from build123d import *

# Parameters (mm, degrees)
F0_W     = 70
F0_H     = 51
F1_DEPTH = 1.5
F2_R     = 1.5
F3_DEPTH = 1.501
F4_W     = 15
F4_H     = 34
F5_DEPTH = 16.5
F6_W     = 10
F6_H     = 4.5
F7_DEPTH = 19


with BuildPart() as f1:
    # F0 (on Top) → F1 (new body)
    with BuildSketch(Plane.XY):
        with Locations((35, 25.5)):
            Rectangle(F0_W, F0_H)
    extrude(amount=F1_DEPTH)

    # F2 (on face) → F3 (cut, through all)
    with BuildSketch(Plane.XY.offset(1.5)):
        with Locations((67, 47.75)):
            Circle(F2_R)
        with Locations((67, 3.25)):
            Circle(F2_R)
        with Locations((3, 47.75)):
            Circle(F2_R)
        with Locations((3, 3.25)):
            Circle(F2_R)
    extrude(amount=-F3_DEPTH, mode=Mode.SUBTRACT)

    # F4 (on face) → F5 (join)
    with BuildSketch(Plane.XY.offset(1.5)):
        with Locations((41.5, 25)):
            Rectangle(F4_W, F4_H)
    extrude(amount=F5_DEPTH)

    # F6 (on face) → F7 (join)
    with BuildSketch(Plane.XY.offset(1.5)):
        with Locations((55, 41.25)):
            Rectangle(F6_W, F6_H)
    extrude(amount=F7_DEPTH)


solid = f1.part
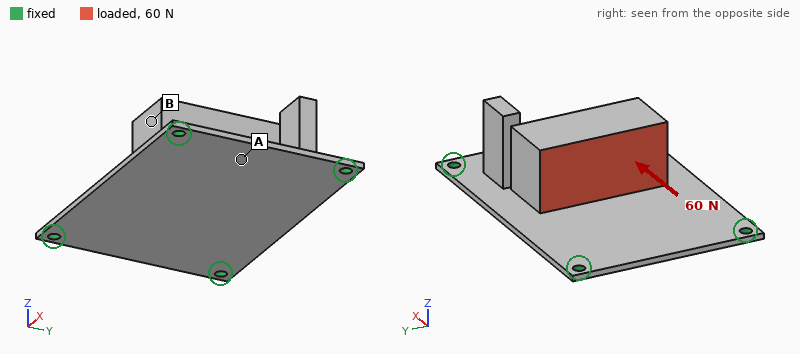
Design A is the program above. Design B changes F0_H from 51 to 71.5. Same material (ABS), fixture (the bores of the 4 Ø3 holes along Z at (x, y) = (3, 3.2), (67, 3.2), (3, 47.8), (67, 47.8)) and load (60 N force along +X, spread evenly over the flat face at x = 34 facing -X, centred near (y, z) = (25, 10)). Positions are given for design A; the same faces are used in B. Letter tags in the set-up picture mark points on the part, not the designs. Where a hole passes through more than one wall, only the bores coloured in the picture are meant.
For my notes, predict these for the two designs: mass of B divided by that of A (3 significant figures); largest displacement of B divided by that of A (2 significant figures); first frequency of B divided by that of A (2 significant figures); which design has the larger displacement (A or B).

1.15
0.81
1.1
A
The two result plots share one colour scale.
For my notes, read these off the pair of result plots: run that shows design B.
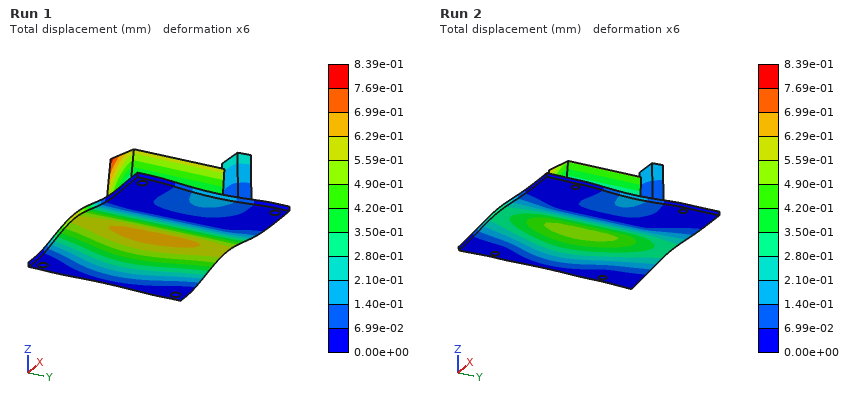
Run 2
